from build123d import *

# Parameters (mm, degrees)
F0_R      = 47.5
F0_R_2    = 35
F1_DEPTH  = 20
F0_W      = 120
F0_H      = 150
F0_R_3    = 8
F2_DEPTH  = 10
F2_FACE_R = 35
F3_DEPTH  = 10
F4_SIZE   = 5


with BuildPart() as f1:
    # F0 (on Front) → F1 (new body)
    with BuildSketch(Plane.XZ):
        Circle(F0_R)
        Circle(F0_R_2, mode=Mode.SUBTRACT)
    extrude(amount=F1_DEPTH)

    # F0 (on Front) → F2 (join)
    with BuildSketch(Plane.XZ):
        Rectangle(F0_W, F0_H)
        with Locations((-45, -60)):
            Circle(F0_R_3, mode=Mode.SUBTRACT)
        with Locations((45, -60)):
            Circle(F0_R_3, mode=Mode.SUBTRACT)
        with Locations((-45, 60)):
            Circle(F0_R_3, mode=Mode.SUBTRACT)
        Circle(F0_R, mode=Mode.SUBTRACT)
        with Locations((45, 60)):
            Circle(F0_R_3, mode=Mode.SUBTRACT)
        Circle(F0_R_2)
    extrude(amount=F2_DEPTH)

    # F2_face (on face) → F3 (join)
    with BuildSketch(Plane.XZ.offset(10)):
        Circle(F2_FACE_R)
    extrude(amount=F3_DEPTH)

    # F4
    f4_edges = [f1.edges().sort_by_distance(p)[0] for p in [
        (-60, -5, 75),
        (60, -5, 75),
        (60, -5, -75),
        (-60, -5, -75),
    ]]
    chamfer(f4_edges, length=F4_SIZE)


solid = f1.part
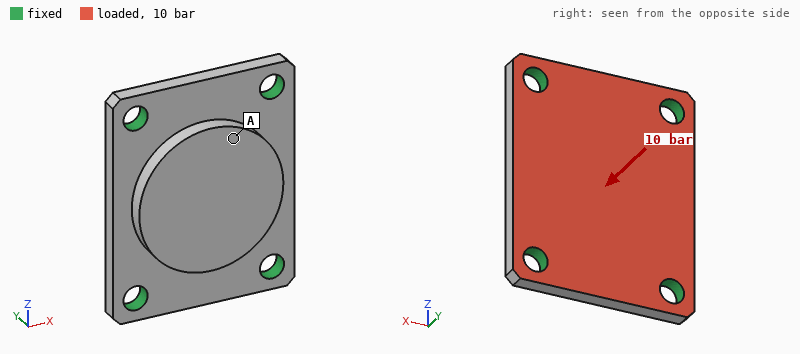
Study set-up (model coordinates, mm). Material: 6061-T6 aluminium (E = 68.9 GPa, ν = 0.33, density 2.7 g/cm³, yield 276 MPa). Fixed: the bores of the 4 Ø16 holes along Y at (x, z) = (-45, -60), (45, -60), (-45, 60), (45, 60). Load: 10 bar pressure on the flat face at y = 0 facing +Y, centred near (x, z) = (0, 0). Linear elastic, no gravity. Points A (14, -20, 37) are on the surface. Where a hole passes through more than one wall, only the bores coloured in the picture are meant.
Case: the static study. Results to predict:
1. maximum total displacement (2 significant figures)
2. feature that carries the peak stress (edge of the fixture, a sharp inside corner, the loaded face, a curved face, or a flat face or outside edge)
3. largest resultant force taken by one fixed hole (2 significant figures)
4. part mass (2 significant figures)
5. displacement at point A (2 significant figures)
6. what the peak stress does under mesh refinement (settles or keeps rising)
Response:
49 µm
edge of the fixture
4.5 kN
650 g
33 µm
keeps rising
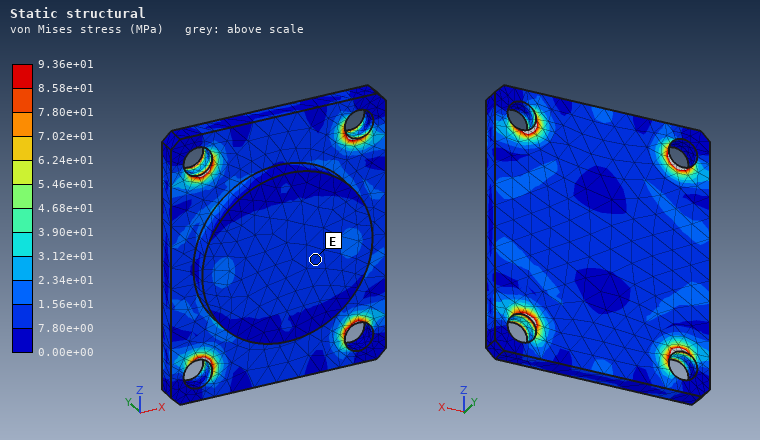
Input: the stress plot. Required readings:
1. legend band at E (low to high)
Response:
7.80e+00 to 1.56e+01 MPa
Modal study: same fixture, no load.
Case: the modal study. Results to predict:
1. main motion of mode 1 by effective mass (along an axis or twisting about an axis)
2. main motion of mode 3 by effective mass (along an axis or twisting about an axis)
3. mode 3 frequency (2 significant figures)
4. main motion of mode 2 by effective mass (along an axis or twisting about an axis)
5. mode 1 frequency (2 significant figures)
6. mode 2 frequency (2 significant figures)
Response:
along Y
twisting about X
7400 Hz
twisting about Z
3900 Hz
5200 Hz
